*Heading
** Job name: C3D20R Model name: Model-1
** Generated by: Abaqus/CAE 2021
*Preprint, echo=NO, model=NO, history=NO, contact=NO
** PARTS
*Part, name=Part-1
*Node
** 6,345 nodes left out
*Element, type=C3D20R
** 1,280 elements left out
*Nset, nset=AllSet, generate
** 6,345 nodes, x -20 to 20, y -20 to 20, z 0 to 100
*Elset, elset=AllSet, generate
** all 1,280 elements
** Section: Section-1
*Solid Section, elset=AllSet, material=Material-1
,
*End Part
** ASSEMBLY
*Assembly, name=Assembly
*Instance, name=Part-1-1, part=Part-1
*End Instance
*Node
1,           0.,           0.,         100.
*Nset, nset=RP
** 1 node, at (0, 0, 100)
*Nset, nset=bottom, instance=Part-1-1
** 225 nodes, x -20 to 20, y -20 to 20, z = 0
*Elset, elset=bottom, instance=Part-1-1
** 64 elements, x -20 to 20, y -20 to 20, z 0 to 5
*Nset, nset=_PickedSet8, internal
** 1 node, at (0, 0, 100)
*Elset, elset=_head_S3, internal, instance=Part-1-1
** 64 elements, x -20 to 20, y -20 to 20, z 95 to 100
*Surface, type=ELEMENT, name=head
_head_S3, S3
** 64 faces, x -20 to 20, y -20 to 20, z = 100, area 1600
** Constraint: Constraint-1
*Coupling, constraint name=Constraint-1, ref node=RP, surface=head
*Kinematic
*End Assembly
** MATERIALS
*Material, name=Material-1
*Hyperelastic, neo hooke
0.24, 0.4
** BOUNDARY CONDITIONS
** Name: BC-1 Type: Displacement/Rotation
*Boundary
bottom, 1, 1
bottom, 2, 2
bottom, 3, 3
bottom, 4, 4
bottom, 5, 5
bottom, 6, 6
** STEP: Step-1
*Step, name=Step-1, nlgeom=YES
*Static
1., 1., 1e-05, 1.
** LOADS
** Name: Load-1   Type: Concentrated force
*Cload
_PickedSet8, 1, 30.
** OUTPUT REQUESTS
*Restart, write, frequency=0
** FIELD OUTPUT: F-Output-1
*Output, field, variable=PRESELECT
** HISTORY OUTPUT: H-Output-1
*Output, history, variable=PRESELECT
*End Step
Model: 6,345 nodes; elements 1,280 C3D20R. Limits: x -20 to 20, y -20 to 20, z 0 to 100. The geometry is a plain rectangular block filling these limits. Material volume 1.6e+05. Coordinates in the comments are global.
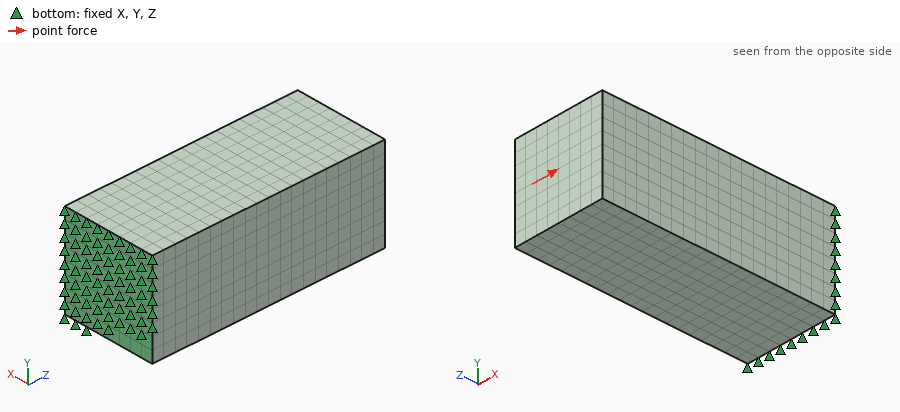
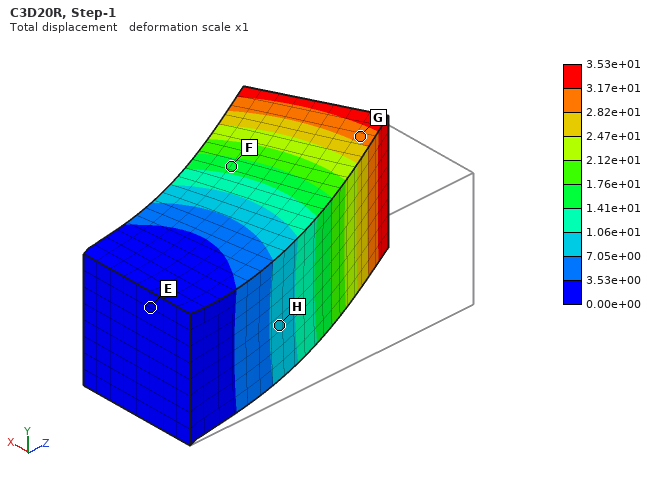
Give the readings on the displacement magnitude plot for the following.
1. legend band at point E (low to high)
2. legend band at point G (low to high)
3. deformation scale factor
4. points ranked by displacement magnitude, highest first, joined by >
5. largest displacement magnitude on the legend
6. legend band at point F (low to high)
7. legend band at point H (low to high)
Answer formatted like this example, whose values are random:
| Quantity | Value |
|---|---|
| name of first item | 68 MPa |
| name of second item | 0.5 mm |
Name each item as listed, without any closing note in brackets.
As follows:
| Quantity | Value |
|---|---|
| legend band at point E | 0.00e+00 to 3.53e+00 |
| legend band at point G | 2.82e+01 to 3.17e+01 |
| deformation scale factor | 1 |
| points ranked by displacement magnitude, highest first, joined by > | G > F > H > E |
| largest displacement magnitude on the legend | 3.53e+01 |
| legend band at point F | 1.41e+01 to 1.76e+01 |
| legend band at point H | 7.05e+00 to 1.06e+01 |
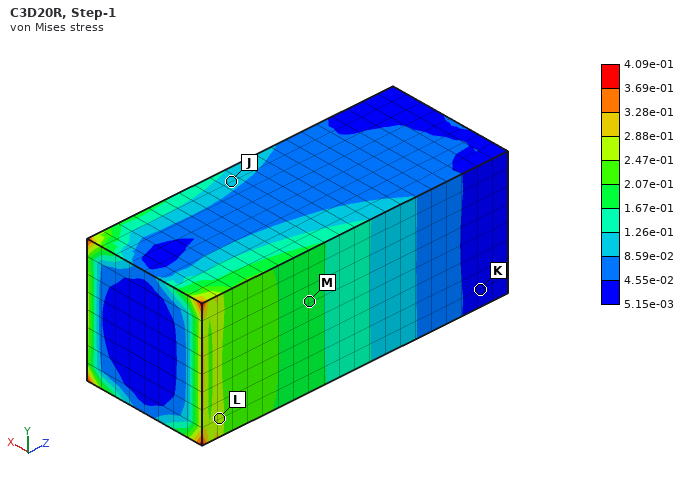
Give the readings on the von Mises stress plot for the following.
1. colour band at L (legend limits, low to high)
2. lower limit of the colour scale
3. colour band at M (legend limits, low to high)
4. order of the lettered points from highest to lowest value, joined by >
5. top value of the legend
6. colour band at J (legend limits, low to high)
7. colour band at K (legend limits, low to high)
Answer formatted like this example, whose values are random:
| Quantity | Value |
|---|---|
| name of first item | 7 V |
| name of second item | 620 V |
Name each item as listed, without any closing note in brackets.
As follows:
| Quantity | Value |
|---|---|
| colour band at L | 2.47e-01 to 2.88e-01 |
| lower limit of the colour scale | 5.15e-03 |
| colour band at M | 1.67e-01 to 2.07e-01 |
| order of the lettered points from highest to lowest value, joined by > | L > M > J > K |
| top value of the legend | 4.09e-01 |
| colour band at J | 8.59e-02 to 1.26e-01 |
| colour band at K | 5.15e-03 to 4.55e-02 |
